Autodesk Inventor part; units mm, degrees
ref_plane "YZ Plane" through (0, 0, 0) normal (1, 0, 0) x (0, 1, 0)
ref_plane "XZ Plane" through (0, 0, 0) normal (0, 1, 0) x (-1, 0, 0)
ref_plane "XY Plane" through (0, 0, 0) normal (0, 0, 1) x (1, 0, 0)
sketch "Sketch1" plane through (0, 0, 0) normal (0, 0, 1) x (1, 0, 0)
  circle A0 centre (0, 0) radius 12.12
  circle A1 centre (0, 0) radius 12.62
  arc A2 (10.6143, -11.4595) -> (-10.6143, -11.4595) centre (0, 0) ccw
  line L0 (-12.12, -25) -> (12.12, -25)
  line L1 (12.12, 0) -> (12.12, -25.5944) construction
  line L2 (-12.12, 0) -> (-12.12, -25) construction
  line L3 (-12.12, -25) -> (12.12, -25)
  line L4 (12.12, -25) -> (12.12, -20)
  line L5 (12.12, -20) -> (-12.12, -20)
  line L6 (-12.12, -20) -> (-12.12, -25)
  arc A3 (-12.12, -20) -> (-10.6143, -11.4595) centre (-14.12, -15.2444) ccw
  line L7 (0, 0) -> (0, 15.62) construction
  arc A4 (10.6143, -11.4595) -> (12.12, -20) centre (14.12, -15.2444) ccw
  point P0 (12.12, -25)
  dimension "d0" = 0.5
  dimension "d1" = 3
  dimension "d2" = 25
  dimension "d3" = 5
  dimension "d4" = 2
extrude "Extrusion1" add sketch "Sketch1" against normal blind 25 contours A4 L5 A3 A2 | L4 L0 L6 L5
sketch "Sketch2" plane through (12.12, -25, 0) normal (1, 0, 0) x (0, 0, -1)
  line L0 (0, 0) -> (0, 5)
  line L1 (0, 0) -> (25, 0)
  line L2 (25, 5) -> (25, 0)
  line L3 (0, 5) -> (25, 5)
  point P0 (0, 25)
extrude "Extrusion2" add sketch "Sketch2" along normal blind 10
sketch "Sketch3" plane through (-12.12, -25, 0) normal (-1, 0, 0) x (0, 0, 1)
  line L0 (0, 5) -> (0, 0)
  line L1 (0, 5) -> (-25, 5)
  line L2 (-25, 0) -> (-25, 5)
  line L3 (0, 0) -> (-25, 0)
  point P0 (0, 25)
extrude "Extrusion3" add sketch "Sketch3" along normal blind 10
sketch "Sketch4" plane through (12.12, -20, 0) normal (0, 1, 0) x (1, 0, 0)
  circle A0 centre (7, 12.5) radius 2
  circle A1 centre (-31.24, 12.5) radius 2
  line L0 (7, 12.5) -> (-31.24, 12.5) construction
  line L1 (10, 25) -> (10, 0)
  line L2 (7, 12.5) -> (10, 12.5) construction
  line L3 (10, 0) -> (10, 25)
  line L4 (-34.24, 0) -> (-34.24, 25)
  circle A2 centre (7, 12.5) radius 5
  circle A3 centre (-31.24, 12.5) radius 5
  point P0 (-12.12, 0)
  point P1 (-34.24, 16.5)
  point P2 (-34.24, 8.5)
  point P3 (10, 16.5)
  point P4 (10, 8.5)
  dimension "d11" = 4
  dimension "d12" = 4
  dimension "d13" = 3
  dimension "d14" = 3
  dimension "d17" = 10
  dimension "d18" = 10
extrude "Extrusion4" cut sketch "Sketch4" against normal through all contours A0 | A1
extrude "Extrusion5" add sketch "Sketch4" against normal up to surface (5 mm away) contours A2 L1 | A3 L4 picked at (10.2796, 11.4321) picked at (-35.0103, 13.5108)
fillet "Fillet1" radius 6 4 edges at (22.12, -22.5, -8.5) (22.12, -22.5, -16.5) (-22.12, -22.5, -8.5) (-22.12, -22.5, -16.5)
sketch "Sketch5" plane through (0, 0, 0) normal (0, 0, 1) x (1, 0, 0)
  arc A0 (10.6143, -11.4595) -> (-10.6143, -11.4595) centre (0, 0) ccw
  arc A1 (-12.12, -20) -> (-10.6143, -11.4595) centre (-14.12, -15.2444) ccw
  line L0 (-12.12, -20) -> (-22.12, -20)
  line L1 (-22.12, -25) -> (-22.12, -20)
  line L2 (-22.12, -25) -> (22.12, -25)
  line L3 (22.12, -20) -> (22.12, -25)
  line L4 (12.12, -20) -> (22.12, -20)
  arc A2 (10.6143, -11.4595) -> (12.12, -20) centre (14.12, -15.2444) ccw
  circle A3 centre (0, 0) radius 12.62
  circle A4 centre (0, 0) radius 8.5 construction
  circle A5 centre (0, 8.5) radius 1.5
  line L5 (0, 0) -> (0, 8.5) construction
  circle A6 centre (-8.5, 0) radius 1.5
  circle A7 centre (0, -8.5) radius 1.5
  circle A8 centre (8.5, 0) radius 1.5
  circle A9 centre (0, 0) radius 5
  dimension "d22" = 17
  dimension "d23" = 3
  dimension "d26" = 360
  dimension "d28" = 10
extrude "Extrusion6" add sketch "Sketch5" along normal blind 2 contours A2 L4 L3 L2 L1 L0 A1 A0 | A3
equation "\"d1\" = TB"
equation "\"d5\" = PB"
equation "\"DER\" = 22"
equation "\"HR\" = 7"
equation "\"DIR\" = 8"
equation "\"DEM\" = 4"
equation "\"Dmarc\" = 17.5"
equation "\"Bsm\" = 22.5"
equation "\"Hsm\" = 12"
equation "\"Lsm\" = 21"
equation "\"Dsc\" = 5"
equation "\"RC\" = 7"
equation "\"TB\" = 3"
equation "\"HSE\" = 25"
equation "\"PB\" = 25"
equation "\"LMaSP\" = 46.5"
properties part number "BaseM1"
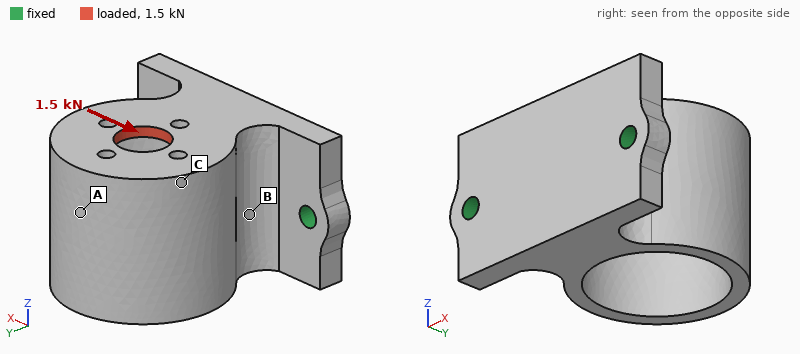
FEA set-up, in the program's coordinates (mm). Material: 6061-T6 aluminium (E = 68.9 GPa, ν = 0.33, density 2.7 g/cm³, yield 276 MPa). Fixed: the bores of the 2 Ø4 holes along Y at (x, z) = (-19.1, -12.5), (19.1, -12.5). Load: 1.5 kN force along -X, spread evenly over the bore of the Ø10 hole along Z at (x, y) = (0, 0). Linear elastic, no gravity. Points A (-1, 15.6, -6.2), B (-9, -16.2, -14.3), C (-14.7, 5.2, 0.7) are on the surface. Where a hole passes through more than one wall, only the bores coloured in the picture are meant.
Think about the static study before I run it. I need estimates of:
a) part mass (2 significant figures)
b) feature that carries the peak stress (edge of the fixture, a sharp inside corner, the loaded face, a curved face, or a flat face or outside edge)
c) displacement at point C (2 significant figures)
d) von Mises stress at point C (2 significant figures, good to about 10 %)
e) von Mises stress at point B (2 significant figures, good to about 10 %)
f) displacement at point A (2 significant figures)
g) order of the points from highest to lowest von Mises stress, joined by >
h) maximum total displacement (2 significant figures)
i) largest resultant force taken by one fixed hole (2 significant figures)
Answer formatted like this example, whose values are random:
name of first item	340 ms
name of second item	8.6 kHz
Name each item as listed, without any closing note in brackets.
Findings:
part mass	45 g
feature that carries the peak stress	a curved face
displacement at point C	0.092 mm
von Mises stress at point C	26 MPa
von Mises stress at point B	38 MPa
displacement at point A	0.11 mm
order of the points from highest to lowest von Mises stress, joined by >	B > C > A
maximum total displacement	0.11 mm
largest resultant force taken by one fixed hole	1.4 kN
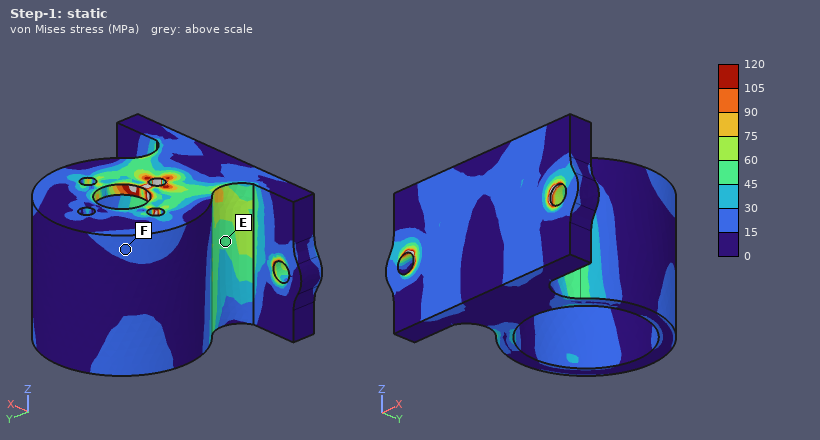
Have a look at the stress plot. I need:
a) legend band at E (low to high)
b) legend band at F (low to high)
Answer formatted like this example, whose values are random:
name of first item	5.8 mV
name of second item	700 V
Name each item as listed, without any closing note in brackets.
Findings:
legend band at E	45 to 60 MPa
legend band at F	15 to 30 MPa
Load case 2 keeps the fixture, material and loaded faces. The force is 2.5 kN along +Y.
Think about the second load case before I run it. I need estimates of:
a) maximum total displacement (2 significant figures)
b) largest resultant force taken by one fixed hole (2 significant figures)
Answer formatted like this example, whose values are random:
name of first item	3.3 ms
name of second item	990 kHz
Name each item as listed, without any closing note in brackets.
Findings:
maximum total displacement	0.29 mm
largest resultant force taken by one fixed hole	1.4 kN
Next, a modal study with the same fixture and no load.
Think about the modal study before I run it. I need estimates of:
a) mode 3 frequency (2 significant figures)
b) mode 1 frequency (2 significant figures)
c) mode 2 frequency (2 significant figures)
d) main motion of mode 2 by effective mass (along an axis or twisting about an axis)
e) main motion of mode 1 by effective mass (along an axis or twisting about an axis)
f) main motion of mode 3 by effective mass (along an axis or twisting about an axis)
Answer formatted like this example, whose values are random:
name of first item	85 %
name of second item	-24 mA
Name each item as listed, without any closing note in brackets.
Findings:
mode 3 frequency	8200 Hz
mode 1 frequency	2700 Hz
mode 2 frequency	4200 Hz
main motion of mode 2 by effective mass	along X
main motion of mode 1 by effective mass	along Z
main motion of mode 3 by effective mass	along Y
